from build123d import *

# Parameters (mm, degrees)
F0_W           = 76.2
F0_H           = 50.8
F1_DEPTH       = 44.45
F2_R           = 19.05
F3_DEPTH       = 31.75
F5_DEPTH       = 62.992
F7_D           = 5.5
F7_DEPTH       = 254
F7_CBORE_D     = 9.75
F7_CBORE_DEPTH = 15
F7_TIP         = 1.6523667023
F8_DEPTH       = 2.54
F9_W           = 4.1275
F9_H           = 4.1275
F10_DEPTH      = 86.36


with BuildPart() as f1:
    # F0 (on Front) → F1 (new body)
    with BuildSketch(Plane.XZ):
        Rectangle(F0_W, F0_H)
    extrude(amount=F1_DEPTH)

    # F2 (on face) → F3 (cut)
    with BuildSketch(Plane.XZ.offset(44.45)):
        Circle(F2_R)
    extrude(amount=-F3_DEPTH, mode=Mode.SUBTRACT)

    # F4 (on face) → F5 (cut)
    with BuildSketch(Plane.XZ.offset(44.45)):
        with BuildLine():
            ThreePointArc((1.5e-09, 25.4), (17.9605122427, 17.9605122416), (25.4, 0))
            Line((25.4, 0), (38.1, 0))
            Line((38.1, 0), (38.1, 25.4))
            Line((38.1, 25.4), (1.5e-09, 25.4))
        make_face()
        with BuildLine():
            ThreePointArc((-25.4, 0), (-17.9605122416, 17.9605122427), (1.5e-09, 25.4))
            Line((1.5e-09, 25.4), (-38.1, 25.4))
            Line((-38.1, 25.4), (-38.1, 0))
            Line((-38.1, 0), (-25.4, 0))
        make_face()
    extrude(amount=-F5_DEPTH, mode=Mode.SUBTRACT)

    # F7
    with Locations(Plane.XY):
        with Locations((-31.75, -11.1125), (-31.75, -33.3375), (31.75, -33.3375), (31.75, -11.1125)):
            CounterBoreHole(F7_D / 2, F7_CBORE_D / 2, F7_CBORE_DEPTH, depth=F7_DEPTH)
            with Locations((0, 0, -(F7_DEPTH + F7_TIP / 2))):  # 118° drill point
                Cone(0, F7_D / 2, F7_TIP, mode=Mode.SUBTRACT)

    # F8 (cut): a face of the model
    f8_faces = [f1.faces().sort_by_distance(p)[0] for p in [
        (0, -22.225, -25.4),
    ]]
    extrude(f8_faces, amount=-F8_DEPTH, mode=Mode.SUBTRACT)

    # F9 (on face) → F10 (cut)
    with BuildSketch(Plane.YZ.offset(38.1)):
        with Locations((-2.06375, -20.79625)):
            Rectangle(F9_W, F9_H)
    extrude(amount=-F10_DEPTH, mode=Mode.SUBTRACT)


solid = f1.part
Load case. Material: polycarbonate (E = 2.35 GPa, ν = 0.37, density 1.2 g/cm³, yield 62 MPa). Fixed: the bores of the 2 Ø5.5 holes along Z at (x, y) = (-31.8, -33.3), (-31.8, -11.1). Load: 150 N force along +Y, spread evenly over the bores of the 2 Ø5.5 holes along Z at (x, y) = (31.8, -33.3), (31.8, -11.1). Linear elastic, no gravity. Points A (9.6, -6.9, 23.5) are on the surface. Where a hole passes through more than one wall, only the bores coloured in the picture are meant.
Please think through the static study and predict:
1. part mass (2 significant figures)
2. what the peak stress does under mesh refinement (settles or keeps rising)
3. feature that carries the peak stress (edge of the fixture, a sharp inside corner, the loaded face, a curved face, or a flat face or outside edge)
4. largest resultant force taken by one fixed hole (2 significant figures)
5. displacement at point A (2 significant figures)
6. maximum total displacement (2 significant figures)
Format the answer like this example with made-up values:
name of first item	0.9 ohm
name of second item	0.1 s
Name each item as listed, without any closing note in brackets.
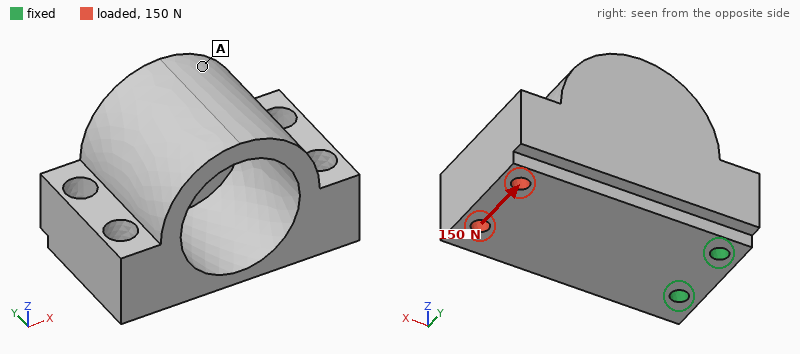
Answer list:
part mass	96 g
what the peak stress does under mesh refinement	keeps rising
feature that carries the peak stress	edge of the fixture
largest resultant force taken by one fixed hole	370 N
displacement at point A	0.067 mm
maximum total displacement	0.20 mm
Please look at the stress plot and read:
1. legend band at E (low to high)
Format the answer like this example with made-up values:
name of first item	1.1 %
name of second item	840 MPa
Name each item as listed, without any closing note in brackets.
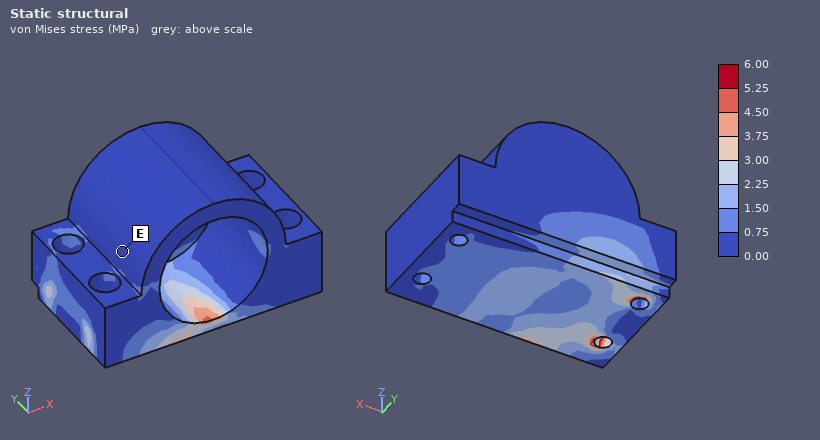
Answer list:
legend band at E	0.00 to 0.75 MPa
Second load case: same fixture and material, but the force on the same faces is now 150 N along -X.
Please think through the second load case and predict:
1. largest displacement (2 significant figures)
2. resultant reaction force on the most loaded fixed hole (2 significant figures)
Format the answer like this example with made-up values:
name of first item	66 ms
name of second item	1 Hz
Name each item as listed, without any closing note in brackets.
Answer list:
largest displacement	26 µm
resultant reaction force on the most loaded fixed hole	75 N
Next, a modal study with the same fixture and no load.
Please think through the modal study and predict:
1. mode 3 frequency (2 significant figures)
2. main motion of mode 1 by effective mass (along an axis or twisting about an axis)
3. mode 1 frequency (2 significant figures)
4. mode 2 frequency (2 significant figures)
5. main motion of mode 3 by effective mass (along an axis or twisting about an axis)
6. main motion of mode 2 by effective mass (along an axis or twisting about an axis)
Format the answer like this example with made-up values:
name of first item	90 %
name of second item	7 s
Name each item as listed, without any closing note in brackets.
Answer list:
mode 3 frequency	1400 Hz
main motion of mode 1 by effective mass	along Z
mode 1 frequency	360 Hz
mode 2 frequency	830 Hz
main motion of mode 3 by effective mass	twisting about X
main motion of mode 2 by effective mass	along Y
